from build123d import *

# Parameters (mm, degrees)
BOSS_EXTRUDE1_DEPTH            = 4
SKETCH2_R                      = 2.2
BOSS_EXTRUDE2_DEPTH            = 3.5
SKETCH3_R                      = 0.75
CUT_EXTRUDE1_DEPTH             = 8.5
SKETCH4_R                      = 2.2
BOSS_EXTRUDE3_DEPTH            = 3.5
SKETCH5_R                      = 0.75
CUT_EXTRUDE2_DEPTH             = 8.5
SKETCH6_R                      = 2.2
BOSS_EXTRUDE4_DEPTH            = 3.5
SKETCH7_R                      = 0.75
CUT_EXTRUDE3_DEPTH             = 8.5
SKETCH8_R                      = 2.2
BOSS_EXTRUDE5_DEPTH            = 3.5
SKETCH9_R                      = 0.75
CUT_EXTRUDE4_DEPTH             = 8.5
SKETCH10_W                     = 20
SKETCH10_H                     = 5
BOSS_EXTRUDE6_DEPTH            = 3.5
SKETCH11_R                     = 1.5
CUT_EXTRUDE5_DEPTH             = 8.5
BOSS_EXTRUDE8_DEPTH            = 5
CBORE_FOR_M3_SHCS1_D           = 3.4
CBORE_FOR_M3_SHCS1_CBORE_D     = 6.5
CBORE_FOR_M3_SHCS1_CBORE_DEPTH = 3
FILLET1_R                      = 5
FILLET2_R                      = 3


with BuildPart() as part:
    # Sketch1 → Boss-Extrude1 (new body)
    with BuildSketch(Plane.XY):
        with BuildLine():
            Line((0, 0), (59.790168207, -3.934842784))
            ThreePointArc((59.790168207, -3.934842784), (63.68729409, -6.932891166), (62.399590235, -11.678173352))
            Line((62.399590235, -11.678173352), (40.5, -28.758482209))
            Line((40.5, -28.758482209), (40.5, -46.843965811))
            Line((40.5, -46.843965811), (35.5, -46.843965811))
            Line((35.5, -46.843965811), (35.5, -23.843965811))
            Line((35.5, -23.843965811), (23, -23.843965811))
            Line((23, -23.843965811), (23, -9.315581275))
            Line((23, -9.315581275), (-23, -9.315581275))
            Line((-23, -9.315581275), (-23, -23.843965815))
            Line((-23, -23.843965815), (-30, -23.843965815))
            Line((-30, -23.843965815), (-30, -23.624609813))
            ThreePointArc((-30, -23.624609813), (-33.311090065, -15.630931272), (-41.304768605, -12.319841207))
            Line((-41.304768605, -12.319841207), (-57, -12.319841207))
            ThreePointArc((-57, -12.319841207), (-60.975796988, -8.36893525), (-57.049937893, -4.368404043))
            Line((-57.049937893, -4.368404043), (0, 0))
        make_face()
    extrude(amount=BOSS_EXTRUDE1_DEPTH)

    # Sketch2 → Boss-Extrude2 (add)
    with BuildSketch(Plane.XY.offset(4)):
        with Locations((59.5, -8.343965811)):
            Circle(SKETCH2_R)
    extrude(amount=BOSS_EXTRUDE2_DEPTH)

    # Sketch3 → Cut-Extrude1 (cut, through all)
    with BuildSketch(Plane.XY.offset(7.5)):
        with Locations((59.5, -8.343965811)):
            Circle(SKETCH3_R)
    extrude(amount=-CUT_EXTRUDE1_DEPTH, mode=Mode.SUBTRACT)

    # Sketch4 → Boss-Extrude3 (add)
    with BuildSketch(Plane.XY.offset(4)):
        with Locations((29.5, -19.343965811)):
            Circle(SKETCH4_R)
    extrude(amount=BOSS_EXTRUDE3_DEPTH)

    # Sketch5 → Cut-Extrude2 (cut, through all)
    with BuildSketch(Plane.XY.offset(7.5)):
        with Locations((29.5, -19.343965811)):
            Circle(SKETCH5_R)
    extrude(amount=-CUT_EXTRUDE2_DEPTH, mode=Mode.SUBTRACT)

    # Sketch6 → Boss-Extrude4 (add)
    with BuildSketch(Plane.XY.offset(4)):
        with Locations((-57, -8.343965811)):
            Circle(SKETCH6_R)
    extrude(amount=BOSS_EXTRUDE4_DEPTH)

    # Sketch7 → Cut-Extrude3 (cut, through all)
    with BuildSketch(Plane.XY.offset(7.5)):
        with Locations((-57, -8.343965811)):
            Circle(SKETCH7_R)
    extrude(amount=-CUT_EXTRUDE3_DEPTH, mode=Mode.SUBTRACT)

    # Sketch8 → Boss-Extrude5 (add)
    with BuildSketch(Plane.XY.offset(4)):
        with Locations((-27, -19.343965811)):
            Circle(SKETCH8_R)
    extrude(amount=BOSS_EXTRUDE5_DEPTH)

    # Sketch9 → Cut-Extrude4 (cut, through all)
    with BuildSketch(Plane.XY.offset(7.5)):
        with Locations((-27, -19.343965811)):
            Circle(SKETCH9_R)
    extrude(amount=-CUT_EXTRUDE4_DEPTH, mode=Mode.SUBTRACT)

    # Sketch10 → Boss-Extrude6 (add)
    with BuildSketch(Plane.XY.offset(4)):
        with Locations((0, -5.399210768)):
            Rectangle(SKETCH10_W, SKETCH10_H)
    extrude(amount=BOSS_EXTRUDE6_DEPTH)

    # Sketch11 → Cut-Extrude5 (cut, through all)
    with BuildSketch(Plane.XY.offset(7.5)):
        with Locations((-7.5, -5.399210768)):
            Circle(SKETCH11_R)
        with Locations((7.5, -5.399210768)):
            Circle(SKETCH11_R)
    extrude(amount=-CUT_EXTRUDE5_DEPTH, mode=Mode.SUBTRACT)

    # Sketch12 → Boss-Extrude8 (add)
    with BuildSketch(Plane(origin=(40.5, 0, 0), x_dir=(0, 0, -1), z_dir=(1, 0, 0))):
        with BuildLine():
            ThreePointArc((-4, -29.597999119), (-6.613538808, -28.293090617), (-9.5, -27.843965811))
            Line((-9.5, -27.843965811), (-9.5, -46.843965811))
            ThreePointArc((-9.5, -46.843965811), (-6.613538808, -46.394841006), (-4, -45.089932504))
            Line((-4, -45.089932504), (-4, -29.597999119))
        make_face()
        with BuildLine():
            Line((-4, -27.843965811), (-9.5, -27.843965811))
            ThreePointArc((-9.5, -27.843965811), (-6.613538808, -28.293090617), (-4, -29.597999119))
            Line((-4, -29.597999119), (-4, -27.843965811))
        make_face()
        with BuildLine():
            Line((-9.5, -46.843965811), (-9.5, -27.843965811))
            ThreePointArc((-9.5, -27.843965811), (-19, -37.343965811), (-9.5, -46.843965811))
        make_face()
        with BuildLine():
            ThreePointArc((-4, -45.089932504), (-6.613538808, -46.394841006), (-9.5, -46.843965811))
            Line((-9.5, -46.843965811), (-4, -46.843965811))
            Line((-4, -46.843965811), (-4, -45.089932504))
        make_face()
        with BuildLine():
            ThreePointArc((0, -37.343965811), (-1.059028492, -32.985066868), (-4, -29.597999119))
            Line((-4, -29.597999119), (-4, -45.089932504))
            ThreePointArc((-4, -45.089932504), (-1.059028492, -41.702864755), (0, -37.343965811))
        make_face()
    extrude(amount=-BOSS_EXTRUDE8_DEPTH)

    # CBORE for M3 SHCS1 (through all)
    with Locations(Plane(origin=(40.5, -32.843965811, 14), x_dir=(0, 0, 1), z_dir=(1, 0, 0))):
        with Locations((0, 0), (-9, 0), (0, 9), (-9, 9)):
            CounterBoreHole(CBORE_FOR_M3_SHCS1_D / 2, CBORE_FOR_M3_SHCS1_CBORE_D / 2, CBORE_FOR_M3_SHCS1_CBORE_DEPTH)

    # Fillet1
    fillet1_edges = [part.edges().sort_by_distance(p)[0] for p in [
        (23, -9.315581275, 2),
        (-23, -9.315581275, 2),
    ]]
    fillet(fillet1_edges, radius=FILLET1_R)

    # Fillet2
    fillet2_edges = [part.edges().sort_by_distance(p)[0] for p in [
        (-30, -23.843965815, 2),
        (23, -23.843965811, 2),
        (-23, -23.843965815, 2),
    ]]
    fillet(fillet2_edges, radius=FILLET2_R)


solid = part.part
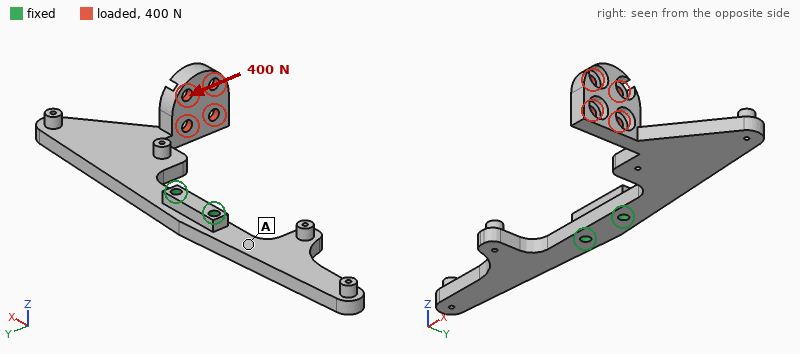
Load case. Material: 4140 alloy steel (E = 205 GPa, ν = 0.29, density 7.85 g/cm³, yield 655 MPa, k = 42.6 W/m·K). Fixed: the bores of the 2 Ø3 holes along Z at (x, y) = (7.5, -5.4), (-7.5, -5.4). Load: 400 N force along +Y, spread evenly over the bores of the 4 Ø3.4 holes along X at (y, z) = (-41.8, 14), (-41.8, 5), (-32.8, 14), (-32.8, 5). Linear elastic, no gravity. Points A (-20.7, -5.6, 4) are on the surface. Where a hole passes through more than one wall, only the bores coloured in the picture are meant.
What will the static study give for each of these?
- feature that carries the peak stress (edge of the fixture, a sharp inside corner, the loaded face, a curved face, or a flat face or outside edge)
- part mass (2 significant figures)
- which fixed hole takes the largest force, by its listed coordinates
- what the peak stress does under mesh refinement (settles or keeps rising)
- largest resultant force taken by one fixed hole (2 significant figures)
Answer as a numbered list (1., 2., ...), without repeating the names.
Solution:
1. edge of the fixture
2. 63 g
3. (7.5, -5.4)
4. keeps rising
5. 750 N
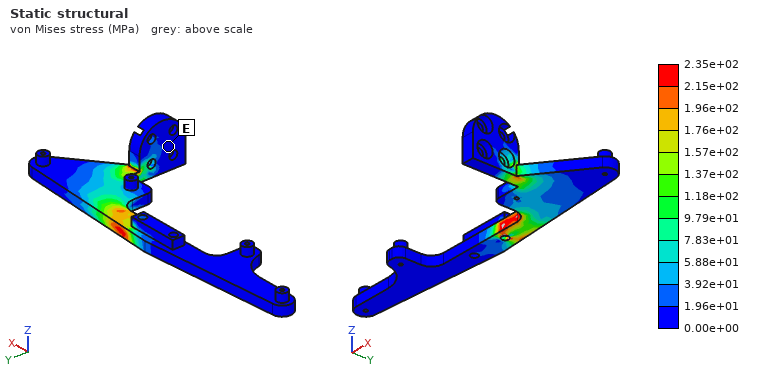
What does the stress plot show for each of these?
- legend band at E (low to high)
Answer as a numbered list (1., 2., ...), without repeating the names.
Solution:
1. 0.00e+00 to 1.96e+01 MPa
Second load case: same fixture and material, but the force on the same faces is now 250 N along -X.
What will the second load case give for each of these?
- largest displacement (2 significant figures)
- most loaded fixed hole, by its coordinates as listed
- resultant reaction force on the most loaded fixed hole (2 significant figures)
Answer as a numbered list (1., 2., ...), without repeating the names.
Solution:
1. 0.34 mm
2. (7.5, -5.4)
3. 440 N
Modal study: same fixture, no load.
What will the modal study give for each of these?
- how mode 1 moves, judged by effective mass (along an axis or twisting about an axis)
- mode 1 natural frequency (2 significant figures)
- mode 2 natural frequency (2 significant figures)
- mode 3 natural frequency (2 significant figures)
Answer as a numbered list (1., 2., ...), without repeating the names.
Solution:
1. along Z
2. 660 Hz
3. 1100 Hz
4. 1200 Hz
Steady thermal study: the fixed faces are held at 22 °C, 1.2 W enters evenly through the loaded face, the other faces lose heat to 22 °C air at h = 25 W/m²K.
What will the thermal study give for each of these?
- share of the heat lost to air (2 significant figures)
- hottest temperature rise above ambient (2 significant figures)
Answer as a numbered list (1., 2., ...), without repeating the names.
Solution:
1. 68 %
2. 19 K
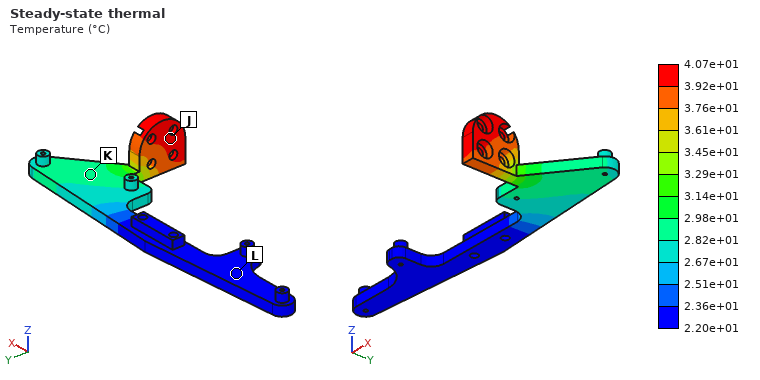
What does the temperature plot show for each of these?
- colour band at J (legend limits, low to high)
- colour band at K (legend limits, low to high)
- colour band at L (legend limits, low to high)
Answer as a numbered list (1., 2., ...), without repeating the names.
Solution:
1. 3.92e+01 to 4.07e+01 °C
2. 2.82e+01 to 2.98e+01 °C
3. 2.20e+01 to 2.36e+01 °C
